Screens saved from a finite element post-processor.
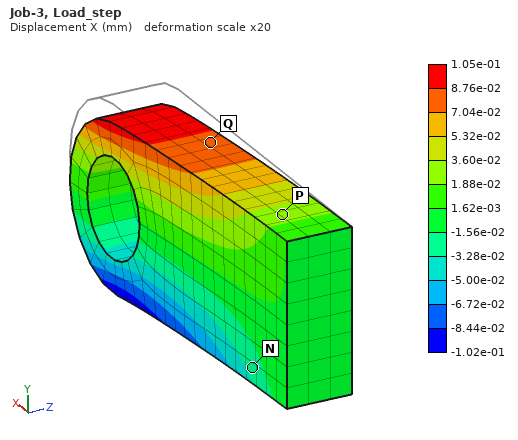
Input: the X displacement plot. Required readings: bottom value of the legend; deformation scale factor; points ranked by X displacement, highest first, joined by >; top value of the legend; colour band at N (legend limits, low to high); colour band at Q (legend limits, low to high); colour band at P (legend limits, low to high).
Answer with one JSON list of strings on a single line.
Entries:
["-1.02e-01 mm", "20", "Q > P > N", "1.05e-01 mm", "-3.28e-02 to -1.56e-02 mm", "7.04e-02 to 8.76e-02 mm", "1.88e-02 to 3.60e-02 mm"]
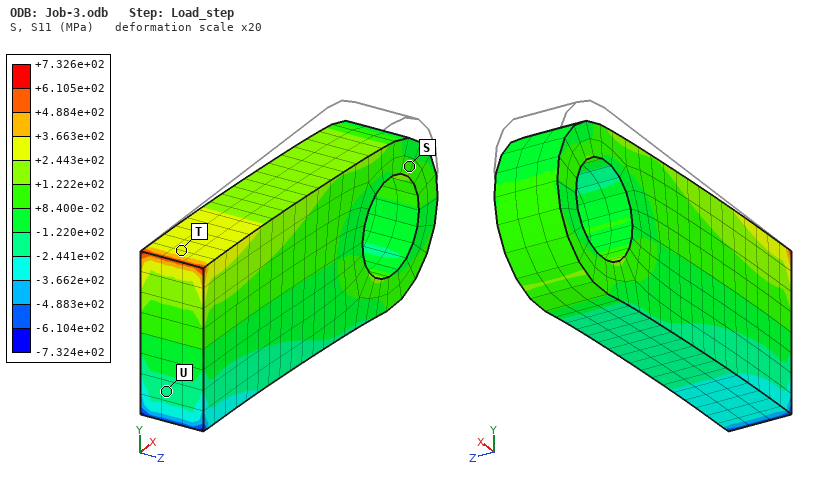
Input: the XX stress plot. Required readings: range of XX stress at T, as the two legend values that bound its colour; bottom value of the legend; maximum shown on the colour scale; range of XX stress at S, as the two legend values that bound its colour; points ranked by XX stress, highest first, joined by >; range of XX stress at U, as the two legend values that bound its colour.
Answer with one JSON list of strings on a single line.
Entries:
["+2.443e+02 to +3.663e+02 MPa", "-7.324e+02 MPa", "+7.326e+02 MPa", "+8.400e-02 to +1.222e+02 MPa", "T > S > U", "-2.441e+02 to -1.220e+02 MPa"]
